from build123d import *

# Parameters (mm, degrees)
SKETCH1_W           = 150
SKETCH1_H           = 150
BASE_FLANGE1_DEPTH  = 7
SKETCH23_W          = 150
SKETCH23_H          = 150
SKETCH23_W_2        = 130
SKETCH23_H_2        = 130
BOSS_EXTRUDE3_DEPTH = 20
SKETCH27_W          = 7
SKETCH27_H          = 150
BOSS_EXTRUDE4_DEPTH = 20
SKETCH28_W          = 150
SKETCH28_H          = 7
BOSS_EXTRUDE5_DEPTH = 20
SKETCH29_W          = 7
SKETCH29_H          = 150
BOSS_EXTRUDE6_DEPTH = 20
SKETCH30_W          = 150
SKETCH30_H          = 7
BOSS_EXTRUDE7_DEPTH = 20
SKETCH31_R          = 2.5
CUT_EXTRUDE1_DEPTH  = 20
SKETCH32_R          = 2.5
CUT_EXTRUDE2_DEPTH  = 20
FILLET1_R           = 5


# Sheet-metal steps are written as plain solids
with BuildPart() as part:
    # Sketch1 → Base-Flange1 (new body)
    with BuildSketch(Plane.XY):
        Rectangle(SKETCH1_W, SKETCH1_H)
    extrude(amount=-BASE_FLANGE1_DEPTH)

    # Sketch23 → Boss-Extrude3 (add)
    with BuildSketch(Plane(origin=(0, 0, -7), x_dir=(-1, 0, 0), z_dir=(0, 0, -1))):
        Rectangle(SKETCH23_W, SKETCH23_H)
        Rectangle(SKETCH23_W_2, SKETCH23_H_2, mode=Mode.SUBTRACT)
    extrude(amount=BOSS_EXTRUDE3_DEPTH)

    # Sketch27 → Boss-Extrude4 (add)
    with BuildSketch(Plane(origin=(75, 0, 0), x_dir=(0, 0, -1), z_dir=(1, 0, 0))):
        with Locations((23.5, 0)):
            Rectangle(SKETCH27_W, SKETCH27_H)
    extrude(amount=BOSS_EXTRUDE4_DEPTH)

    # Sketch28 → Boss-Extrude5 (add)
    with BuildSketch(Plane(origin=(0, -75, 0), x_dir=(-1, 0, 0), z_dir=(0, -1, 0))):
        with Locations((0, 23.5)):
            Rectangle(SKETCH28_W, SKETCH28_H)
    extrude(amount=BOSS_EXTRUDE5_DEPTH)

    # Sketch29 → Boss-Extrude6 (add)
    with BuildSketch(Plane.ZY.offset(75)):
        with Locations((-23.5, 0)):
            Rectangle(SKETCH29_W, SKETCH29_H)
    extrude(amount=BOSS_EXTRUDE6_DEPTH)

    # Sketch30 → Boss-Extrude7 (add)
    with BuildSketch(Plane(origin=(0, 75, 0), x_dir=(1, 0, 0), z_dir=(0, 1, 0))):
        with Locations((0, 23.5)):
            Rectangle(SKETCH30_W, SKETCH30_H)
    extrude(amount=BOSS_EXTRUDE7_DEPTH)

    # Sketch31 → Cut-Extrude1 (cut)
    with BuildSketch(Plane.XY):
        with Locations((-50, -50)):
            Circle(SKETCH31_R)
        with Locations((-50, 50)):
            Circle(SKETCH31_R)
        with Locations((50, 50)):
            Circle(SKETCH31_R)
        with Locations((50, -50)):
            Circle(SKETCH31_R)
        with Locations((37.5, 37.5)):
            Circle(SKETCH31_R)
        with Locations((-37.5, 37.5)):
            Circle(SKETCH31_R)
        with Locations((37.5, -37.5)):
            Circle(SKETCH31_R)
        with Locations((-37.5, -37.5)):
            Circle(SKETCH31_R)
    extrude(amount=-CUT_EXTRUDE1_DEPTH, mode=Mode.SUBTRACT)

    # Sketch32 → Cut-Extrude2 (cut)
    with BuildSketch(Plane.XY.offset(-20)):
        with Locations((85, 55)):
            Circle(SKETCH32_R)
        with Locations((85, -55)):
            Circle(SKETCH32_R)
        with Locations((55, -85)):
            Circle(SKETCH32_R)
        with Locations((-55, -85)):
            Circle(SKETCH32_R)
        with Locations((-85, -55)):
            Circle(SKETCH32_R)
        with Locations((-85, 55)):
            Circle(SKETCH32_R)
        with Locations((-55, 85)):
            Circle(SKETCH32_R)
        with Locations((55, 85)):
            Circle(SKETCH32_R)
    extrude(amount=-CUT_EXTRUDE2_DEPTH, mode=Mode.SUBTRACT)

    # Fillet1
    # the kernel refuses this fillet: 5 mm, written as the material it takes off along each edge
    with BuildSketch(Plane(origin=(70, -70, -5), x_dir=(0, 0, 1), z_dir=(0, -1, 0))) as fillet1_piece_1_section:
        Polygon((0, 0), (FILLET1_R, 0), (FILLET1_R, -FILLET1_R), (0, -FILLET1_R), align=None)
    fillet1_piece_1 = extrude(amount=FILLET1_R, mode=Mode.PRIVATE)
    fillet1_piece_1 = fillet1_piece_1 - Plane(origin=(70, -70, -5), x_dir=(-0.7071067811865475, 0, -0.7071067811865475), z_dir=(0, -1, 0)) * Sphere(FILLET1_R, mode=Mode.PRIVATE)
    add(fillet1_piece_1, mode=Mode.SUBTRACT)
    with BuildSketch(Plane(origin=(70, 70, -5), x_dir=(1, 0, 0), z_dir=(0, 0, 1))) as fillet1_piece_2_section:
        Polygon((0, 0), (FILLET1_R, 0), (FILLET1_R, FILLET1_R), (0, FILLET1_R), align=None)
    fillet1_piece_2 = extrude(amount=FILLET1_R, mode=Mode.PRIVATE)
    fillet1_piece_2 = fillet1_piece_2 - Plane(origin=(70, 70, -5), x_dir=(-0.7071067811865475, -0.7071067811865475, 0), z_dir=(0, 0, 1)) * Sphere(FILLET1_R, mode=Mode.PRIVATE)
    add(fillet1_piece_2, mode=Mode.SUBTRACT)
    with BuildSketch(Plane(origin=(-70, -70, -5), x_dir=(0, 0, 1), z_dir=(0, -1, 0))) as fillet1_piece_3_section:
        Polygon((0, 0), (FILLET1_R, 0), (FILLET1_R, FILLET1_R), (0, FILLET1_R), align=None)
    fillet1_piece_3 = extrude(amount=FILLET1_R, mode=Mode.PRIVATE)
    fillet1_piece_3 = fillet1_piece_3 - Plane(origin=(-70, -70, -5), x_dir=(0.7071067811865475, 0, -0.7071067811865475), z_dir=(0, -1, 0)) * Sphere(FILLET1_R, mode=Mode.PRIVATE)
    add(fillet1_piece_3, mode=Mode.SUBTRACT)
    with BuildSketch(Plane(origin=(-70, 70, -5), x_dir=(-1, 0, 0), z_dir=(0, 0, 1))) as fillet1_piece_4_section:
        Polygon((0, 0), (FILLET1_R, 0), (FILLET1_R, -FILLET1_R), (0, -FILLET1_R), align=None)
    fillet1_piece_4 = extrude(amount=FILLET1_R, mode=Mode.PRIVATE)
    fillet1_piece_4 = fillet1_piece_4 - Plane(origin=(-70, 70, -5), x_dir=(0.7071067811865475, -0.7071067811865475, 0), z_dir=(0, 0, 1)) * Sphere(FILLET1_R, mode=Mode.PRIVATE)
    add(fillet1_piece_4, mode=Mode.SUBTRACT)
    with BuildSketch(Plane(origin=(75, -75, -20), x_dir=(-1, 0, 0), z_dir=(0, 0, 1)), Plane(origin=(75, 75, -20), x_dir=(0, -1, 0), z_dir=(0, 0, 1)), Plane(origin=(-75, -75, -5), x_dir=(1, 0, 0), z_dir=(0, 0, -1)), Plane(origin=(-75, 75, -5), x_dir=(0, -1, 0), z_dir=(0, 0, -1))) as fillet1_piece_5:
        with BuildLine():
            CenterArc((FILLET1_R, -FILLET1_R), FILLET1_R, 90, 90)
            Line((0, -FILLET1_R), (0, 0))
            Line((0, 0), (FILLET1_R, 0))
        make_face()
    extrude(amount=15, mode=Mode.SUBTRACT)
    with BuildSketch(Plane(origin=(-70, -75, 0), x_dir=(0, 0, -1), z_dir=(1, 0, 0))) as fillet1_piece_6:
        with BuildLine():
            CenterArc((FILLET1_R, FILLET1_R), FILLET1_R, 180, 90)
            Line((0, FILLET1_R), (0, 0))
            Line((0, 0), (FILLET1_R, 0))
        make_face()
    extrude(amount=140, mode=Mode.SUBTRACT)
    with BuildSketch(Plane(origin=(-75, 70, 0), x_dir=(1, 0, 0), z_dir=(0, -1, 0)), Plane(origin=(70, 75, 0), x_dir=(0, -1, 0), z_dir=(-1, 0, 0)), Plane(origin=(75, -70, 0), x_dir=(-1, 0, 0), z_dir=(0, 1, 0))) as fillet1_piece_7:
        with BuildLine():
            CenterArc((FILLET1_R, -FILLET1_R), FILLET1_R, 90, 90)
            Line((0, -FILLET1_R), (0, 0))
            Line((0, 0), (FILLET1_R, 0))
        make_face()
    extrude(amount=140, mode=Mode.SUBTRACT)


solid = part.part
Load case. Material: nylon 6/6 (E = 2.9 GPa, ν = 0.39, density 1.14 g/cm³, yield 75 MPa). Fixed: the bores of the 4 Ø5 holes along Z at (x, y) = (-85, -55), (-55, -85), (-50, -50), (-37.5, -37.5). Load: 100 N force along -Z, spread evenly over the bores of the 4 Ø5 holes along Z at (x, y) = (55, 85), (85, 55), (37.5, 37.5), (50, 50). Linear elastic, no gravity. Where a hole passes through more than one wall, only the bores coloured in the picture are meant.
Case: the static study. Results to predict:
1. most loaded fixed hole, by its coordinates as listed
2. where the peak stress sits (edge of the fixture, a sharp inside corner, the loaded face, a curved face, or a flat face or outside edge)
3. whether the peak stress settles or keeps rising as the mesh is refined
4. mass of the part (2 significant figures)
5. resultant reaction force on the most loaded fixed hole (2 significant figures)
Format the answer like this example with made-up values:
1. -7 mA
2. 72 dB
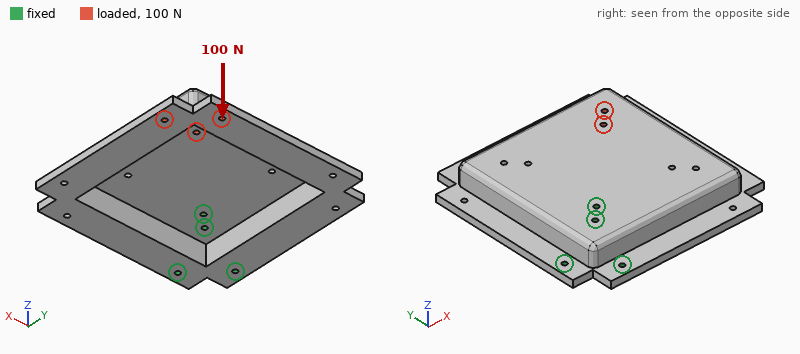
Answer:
1. (-37.5, -37.5)
2. edge of the fixture
3. keeps rising
4. 400 g
5. 290 N
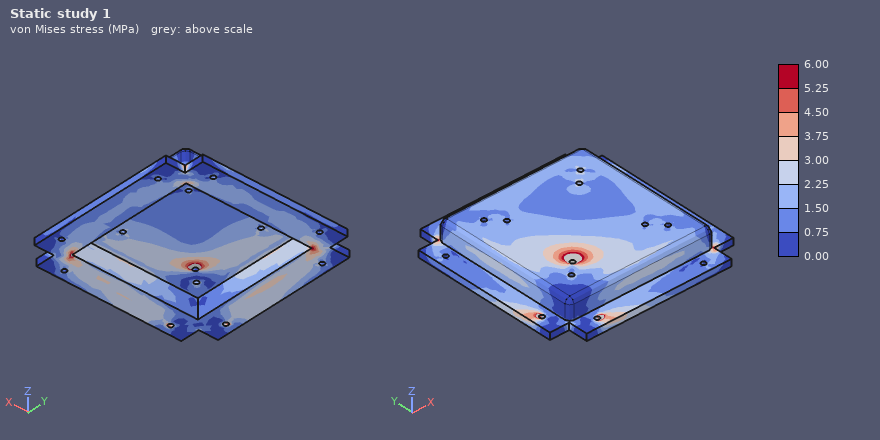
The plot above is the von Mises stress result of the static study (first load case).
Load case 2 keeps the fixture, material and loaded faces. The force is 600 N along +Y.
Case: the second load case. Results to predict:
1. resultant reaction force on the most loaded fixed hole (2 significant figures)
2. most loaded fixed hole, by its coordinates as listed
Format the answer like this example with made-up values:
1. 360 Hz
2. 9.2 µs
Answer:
1. 1.6 kN
2. (-37.5, -37.5)
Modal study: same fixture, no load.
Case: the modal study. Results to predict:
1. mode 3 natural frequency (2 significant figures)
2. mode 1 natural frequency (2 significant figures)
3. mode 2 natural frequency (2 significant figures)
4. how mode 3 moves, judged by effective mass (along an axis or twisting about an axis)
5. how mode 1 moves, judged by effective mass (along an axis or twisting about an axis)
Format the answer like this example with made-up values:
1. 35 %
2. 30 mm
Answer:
1. 330 Hz
2. 110 Hz
3. 170 Hz
4. along Z
5. along Z
